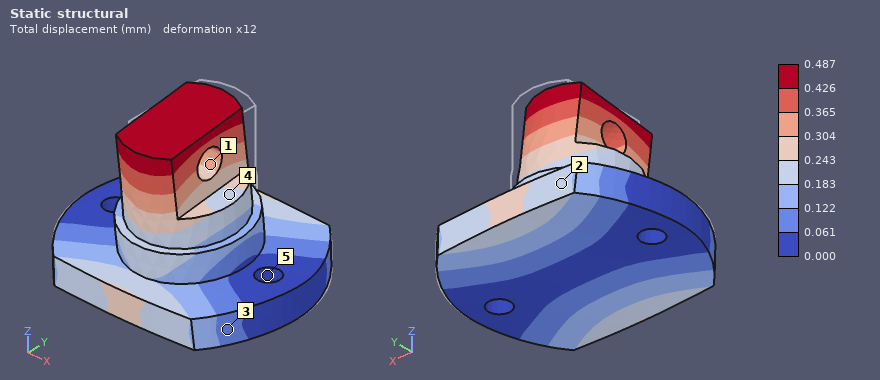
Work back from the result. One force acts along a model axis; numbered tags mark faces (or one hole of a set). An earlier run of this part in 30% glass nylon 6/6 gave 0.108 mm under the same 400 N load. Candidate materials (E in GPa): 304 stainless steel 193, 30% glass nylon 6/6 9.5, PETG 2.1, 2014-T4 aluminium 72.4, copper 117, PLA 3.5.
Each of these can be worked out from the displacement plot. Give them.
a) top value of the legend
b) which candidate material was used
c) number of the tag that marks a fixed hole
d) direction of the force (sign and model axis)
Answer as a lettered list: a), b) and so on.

a) 0.487 mm
b) PETG
c) 5
d) -Y
